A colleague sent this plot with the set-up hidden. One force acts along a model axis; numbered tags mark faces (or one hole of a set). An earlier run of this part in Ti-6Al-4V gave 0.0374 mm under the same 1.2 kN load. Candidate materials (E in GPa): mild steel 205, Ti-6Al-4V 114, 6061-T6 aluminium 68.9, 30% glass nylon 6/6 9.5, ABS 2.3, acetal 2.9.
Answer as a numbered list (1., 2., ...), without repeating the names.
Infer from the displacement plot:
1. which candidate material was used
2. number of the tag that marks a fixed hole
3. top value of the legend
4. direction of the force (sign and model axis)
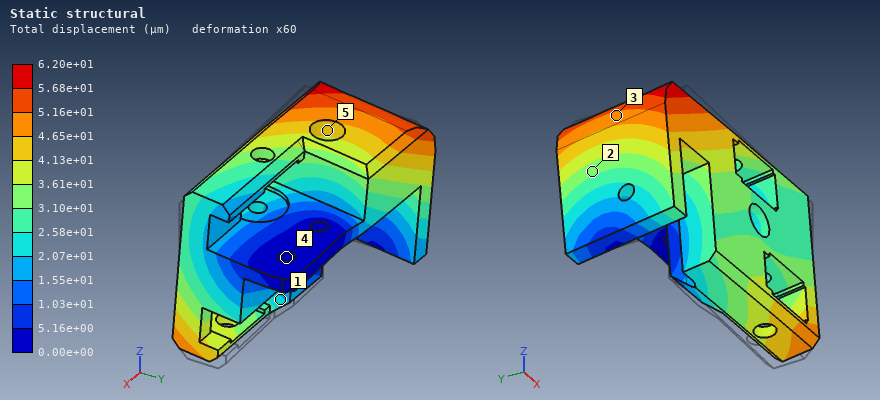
1. 6061-T6 aluminium
2. 4
3. 6.20e+01 µm
4. +Y
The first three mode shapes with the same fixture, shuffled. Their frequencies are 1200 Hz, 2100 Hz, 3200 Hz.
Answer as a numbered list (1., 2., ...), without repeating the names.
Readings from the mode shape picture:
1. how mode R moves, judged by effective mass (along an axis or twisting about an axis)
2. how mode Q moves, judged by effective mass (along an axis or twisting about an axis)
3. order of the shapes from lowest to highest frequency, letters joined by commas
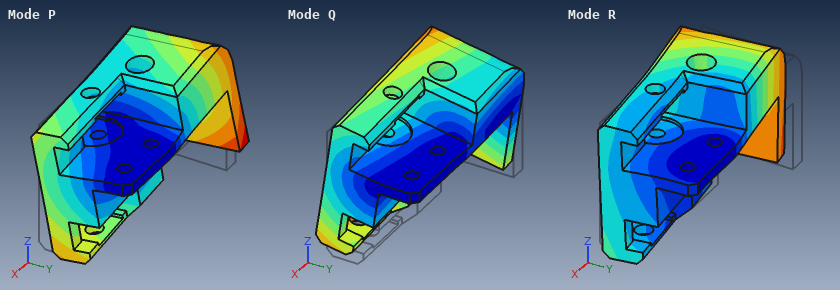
1. along Y
2. along Z
3. Q, P, R
